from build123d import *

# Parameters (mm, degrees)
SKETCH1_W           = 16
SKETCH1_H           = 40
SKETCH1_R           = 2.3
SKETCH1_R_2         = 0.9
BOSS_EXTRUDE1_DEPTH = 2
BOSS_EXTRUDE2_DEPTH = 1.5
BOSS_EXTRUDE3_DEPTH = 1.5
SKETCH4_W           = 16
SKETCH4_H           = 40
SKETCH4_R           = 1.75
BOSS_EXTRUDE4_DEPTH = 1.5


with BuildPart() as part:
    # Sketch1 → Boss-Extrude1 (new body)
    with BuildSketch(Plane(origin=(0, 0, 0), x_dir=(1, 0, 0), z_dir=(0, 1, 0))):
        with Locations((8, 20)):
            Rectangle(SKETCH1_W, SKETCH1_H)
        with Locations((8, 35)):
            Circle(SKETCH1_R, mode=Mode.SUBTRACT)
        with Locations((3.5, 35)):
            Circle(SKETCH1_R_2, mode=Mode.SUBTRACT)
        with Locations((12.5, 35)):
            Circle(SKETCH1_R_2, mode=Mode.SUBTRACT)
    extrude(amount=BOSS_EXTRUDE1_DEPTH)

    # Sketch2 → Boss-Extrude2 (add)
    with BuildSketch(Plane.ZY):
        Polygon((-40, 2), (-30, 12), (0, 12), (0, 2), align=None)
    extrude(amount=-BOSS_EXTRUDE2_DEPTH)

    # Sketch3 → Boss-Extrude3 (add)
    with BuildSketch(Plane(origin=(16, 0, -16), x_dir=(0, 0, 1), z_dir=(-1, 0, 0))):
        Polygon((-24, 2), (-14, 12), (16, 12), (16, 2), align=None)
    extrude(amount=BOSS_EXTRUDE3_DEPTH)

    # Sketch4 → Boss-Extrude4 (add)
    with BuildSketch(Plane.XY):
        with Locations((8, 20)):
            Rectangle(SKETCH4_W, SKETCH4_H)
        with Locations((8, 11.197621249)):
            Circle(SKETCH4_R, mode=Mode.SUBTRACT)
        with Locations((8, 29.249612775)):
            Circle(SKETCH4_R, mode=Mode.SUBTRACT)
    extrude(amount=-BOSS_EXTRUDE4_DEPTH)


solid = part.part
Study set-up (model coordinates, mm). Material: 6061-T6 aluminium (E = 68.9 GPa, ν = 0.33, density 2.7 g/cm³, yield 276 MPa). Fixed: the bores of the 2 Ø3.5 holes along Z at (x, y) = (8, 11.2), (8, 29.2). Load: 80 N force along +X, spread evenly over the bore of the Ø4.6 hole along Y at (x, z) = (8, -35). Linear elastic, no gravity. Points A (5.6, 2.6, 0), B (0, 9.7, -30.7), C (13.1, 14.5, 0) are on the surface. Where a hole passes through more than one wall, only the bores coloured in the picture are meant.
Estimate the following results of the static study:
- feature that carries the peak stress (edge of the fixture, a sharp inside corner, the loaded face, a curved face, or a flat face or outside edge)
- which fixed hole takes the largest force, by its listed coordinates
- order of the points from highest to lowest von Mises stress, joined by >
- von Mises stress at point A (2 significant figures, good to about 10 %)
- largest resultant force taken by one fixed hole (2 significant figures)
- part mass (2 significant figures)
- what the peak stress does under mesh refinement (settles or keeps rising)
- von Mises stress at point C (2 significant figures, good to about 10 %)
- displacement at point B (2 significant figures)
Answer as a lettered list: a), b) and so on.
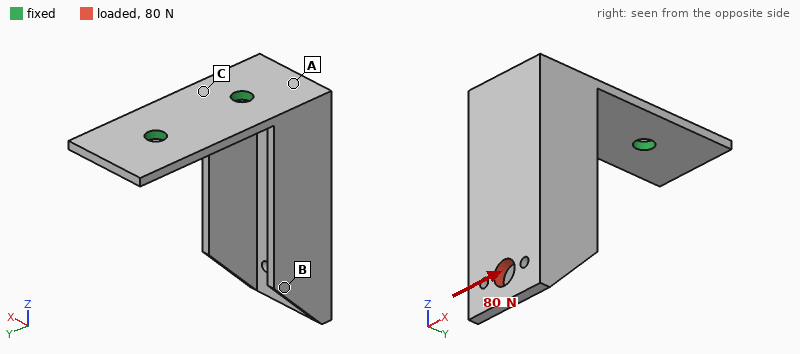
a) edge of the fixture
b) (8, 11.2)
c) C > A > B
d) 50 MPa
e) 110 N
f) 8.4 g
g) keeps rising
h) 110 MPa
i) 0.53 mm
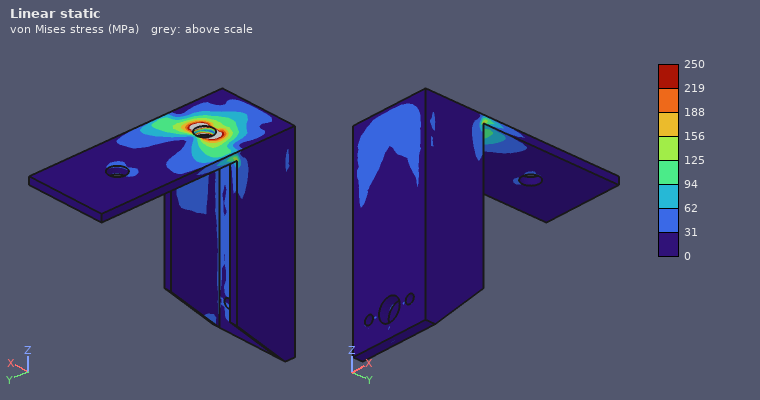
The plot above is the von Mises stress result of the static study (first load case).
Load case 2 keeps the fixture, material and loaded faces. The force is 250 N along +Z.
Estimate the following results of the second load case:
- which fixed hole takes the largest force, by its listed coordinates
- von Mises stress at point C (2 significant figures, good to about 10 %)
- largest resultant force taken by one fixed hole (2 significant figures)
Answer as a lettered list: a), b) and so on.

a) (8, 11.2)
b) 56 MPa
c) 280 N
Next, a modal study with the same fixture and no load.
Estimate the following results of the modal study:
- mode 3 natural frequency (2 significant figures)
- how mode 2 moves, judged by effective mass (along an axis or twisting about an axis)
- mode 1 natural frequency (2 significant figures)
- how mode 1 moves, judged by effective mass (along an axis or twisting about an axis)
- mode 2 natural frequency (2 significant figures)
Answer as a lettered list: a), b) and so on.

a) 4900 Hz
b) along X
c) 1100 Hz
d) along Y
e) 1200 Hz
